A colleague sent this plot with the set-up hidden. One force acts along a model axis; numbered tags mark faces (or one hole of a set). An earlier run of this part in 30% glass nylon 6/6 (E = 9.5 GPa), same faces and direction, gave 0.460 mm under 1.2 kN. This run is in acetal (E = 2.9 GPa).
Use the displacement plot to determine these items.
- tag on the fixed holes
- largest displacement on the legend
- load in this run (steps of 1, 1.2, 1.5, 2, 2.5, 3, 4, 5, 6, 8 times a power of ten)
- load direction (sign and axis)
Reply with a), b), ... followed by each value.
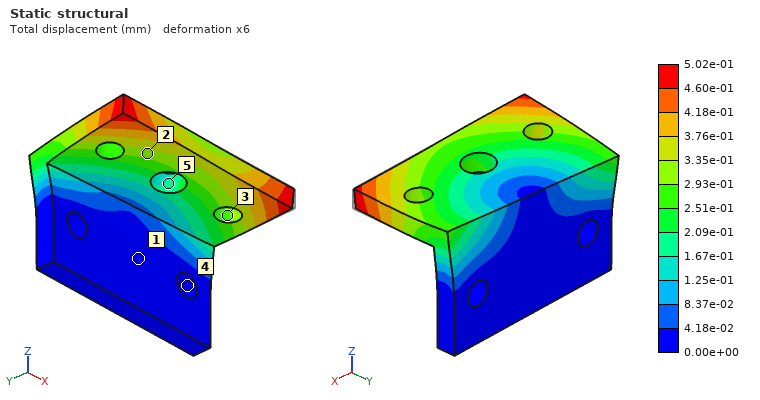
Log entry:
a) 4
b) 5.02e-01 mm
c) 400 N
d) -X
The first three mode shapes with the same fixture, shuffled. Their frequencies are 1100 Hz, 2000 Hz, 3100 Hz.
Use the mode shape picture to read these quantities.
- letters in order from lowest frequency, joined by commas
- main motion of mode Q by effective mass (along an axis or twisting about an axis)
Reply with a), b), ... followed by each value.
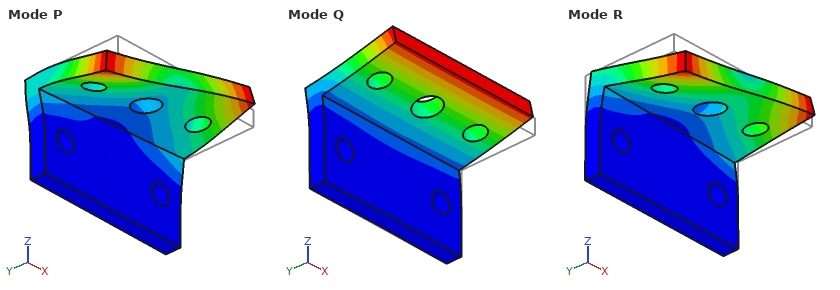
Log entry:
a) Q, R, P
b) along Z
